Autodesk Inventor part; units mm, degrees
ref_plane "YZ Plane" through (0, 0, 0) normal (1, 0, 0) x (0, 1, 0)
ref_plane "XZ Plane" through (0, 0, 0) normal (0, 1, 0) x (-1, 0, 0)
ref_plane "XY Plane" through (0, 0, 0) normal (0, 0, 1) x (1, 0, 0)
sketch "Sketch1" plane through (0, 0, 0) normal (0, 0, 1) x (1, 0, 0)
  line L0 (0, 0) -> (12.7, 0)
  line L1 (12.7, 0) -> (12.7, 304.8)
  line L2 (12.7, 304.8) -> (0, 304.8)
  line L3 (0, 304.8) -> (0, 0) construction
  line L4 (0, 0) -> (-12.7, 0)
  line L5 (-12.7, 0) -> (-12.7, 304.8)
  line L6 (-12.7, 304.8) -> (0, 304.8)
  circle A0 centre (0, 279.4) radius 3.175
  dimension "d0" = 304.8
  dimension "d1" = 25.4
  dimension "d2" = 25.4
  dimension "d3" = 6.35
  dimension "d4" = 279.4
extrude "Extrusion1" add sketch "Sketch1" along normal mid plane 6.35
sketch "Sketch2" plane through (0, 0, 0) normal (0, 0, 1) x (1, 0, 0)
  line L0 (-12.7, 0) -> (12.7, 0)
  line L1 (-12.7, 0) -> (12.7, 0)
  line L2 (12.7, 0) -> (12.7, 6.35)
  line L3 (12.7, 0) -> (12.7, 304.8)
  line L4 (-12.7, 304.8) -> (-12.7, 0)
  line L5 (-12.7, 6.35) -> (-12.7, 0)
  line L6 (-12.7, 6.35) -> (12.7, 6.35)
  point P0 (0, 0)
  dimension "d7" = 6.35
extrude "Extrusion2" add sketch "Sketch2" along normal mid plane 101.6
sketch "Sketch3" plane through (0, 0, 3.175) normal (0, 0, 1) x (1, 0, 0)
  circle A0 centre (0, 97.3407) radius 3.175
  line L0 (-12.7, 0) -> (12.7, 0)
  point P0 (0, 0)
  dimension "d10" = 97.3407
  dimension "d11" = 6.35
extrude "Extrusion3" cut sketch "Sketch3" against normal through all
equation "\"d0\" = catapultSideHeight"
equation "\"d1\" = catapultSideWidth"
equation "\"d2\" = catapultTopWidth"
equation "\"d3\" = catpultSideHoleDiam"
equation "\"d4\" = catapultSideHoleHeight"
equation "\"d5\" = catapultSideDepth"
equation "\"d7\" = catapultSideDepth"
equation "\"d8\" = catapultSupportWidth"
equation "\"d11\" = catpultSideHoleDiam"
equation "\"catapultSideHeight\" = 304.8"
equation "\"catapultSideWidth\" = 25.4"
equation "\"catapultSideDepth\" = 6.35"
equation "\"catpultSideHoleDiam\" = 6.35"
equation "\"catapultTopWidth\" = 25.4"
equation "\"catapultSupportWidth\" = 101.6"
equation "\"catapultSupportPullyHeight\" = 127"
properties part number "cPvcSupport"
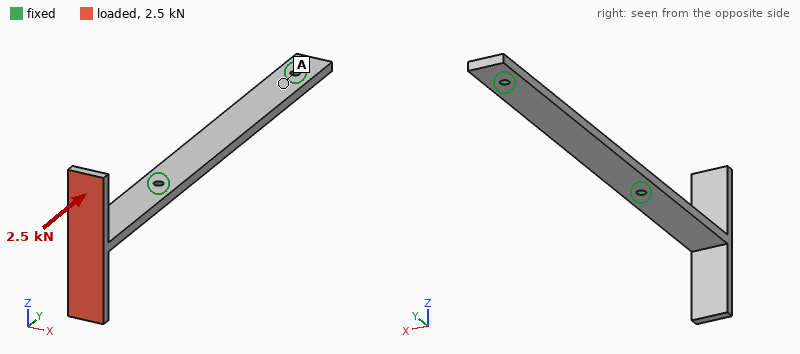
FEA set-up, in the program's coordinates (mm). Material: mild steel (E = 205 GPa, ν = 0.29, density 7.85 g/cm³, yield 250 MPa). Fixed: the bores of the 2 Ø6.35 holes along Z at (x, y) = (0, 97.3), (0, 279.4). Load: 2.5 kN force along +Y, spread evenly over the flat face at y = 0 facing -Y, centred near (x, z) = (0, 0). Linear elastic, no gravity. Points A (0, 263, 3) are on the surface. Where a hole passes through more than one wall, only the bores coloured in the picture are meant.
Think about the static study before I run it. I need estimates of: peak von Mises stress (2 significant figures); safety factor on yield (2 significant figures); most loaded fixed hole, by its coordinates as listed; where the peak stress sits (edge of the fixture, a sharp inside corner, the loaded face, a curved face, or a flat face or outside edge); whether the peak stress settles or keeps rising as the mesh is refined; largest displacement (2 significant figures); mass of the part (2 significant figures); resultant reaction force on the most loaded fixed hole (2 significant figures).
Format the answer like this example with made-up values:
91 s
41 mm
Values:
150 MPa
1.7
(0, 97.3)
the loaded face
settles
0.18 mm
500 g
2.4 kN
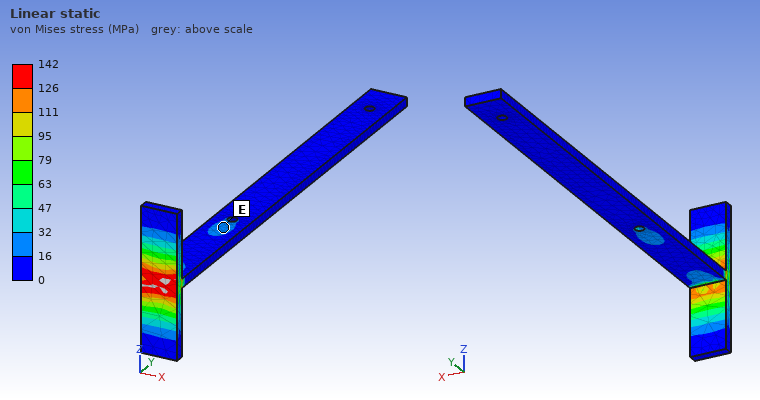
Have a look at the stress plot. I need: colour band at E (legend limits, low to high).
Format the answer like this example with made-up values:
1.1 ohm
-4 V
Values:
16 to 32 MPa
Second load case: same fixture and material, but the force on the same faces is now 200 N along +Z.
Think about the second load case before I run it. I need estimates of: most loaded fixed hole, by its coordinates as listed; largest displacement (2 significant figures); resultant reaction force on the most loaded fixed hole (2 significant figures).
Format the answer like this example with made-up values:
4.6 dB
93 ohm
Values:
(0, 97.3)
0.69 mm
200 N
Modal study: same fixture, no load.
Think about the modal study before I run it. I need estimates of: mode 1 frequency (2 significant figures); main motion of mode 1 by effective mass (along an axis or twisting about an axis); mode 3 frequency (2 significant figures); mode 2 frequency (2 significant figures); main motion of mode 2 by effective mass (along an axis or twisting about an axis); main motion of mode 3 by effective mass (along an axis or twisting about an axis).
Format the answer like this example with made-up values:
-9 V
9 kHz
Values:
240 Hz
along Z
800 Hz
590 Hz
twisting about Y
along X
